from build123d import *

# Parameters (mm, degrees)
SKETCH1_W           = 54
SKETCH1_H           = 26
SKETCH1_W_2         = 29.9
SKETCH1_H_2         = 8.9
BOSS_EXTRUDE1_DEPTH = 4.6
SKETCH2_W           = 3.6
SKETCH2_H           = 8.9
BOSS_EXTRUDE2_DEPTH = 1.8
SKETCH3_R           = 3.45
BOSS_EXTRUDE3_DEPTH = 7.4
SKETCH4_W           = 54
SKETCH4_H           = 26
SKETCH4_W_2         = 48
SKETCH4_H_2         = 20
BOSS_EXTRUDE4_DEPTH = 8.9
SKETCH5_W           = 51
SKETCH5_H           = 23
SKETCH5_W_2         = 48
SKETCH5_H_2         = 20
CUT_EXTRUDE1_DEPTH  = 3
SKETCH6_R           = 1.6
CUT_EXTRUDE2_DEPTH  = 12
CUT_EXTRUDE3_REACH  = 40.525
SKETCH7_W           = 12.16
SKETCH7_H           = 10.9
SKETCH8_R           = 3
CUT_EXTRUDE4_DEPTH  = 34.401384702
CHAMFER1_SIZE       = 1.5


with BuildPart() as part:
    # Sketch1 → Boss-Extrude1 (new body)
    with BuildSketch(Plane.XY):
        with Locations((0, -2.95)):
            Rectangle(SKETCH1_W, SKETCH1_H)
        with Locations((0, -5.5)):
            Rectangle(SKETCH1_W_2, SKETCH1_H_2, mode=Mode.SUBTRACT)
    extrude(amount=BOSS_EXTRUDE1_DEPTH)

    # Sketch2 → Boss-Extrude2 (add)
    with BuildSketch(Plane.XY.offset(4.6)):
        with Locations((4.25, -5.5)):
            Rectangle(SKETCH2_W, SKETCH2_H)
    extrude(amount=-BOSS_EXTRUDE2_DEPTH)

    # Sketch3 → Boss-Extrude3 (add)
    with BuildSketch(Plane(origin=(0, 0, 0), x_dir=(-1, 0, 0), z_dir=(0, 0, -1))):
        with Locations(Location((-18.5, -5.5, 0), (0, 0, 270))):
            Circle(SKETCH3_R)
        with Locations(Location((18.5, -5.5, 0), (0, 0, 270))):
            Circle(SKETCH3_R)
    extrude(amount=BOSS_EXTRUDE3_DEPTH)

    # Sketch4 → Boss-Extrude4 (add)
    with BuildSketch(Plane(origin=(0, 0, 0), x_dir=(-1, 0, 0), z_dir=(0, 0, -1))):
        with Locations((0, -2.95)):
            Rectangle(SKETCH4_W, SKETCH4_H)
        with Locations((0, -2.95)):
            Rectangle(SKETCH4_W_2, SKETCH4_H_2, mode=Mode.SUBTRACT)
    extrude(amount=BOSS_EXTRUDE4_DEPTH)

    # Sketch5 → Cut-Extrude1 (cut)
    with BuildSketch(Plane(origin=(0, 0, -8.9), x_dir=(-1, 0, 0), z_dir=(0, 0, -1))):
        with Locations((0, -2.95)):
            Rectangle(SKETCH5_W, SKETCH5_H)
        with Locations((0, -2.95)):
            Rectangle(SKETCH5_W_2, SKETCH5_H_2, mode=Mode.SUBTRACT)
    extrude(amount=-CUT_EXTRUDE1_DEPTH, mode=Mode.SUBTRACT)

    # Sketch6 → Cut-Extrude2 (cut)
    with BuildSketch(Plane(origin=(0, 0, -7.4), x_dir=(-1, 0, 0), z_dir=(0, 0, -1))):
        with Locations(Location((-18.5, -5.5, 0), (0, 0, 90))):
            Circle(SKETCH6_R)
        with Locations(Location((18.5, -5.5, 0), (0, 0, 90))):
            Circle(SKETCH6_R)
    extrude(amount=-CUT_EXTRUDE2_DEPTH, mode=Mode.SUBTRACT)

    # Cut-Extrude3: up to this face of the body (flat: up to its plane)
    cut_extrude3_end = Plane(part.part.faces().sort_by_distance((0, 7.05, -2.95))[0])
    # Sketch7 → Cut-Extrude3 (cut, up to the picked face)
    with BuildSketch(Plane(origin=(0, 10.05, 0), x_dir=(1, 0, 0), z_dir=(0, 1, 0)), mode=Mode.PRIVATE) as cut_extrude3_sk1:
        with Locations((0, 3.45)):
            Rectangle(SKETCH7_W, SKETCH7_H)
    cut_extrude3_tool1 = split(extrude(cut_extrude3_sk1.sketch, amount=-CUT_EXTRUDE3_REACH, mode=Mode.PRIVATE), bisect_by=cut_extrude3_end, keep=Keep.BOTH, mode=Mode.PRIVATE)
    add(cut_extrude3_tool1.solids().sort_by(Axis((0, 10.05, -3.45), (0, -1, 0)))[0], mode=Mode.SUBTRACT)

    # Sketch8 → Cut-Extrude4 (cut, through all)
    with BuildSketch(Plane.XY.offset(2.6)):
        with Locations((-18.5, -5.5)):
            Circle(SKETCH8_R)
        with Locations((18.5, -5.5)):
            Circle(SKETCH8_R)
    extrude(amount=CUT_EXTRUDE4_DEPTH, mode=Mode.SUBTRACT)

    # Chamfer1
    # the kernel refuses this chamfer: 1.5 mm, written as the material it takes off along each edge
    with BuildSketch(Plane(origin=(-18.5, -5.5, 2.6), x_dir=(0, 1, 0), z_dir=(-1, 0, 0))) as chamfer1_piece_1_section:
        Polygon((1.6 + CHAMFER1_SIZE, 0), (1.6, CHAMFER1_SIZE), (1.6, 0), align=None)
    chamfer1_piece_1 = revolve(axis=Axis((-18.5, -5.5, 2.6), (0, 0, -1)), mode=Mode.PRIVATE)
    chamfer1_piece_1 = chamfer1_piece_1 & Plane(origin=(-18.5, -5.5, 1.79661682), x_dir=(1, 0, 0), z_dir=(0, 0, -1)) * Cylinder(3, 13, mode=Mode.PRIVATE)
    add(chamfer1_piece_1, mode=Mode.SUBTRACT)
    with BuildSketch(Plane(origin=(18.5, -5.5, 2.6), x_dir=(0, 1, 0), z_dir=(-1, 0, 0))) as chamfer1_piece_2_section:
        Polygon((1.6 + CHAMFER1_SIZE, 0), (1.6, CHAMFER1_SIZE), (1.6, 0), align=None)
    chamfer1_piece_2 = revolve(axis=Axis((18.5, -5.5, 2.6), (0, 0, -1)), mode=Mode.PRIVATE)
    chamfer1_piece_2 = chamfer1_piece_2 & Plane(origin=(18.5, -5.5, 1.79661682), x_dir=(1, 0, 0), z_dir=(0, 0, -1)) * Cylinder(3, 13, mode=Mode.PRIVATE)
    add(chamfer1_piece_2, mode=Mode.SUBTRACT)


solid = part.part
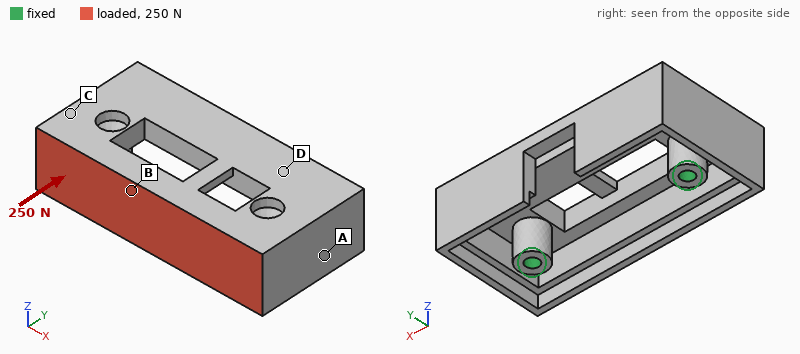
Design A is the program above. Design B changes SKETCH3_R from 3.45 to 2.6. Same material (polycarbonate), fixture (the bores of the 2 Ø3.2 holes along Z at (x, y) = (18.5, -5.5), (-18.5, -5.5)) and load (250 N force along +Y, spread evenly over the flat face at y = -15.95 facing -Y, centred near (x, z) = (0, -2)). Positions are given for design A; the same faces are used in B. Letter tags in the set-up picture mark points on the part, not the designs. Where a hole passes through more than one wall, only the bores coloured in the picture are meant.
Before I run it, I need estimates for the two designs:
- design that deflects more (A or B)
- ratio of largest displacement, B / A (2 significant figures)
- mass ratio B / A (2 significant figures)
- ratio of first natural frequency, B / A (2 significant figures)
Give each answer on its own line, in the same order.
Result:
B
1.2
0.97
0.77
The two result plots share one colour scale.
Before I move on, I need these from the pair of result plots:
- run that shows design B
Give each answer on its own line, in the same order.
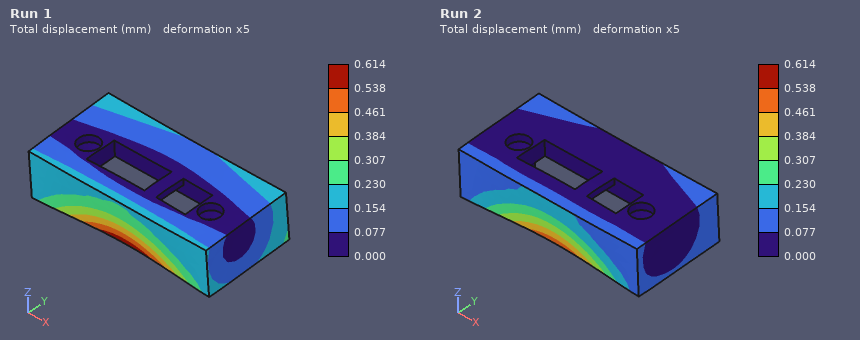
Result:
Run 1
